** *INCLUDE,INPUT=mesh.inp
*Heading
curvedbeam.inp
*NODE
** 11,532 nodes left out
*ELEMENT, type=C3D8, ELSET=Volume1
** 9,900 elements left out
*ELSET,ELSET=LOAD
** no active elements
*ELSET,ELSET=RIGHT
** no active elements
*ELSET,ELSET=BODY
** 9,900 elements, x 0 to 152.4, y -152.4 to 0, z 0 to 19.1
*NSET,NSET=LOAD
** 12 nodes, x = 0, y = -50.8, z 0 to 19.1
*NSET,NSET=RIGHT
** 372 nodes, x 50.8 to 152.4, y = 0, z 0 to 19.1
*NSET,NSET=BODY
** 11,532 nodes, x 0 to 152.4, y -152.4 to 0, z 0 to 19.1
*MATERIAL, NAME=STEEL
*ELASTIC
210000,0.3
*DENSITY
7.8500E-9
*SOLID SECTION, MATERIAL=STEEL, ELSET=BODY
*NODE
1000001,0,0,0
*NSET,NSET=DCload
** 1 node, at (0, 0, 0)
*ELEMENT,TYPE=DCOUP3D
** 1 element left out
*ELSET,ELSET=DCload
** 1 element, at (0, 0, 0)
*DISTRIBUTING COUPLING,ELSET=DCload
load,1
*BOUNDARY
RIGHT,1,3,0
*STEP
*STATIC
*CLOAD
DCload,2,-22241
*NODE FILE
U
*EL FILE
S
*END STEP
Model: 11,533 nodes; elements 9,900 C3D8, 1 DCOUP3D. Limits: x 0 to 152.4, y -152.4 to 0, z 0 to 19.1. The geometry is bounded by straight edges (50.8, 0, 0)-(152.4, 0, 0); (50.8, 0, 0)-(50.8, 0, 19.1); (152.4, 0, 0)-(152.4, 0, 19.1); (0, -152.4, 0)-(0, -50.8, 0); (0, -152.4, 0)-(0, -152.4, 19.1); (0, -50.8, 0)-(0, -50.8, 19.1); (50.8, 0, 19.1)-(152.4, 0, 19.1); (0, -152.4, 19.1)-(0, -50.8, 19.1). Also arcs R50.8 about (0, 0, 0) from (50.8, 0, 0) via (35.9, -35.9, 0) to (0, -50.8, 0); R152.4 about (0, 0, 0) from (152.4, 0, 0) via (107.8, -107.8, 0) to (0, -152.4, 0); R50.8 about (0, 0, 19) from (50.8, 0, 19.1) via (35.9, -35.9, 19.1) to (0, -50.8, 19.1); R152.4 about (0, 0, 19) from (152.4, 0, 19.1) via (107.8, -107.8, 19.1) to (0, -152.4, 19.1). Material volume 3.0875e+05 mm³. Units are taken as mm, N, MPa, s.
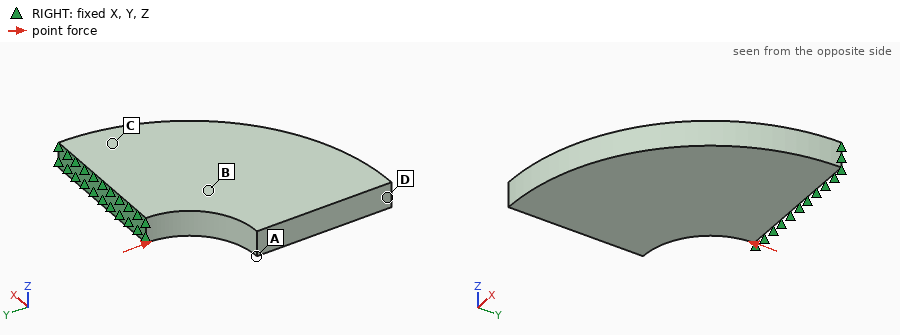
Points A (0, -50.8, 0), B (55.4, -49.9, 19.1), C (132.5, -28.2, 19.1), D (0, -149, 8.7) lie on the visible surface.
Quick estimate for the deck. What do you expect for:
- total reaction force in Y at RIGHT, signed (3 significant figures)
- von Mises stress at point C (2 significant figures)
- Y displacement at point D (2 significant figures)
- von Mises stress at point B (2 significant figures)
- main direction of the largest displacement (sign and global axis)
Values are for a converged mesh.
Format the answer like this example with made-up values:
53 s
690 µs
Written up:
22200 N
31 MPa
-0.053 mm
32 MPa
-Y
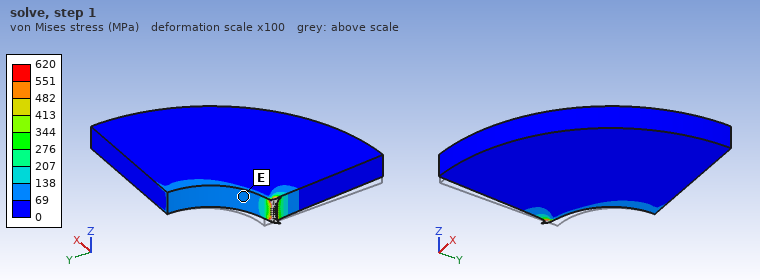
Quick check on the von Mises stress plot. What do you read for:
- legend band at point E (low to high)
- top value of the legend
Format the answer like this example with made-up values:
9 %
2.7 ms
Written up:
69 to 138 MPa
620 MPa
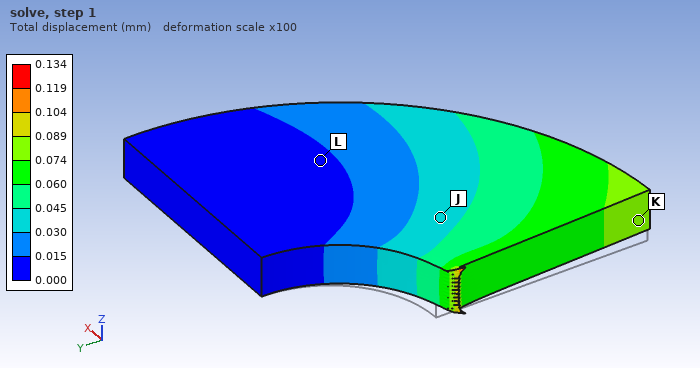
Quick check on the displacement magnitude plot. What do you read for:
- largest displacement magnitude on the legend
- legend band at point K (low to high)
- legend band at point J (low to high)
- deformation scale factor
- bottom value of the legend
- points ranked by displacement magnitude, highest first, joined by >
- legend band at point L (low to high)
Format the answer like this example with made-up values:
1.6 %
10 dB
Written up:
0.134 mm
0.074 to 0.089 mm
0.030 to 0.045 mm
100
0.000 mm
K > J > L
0.000 to 0.015 mm
